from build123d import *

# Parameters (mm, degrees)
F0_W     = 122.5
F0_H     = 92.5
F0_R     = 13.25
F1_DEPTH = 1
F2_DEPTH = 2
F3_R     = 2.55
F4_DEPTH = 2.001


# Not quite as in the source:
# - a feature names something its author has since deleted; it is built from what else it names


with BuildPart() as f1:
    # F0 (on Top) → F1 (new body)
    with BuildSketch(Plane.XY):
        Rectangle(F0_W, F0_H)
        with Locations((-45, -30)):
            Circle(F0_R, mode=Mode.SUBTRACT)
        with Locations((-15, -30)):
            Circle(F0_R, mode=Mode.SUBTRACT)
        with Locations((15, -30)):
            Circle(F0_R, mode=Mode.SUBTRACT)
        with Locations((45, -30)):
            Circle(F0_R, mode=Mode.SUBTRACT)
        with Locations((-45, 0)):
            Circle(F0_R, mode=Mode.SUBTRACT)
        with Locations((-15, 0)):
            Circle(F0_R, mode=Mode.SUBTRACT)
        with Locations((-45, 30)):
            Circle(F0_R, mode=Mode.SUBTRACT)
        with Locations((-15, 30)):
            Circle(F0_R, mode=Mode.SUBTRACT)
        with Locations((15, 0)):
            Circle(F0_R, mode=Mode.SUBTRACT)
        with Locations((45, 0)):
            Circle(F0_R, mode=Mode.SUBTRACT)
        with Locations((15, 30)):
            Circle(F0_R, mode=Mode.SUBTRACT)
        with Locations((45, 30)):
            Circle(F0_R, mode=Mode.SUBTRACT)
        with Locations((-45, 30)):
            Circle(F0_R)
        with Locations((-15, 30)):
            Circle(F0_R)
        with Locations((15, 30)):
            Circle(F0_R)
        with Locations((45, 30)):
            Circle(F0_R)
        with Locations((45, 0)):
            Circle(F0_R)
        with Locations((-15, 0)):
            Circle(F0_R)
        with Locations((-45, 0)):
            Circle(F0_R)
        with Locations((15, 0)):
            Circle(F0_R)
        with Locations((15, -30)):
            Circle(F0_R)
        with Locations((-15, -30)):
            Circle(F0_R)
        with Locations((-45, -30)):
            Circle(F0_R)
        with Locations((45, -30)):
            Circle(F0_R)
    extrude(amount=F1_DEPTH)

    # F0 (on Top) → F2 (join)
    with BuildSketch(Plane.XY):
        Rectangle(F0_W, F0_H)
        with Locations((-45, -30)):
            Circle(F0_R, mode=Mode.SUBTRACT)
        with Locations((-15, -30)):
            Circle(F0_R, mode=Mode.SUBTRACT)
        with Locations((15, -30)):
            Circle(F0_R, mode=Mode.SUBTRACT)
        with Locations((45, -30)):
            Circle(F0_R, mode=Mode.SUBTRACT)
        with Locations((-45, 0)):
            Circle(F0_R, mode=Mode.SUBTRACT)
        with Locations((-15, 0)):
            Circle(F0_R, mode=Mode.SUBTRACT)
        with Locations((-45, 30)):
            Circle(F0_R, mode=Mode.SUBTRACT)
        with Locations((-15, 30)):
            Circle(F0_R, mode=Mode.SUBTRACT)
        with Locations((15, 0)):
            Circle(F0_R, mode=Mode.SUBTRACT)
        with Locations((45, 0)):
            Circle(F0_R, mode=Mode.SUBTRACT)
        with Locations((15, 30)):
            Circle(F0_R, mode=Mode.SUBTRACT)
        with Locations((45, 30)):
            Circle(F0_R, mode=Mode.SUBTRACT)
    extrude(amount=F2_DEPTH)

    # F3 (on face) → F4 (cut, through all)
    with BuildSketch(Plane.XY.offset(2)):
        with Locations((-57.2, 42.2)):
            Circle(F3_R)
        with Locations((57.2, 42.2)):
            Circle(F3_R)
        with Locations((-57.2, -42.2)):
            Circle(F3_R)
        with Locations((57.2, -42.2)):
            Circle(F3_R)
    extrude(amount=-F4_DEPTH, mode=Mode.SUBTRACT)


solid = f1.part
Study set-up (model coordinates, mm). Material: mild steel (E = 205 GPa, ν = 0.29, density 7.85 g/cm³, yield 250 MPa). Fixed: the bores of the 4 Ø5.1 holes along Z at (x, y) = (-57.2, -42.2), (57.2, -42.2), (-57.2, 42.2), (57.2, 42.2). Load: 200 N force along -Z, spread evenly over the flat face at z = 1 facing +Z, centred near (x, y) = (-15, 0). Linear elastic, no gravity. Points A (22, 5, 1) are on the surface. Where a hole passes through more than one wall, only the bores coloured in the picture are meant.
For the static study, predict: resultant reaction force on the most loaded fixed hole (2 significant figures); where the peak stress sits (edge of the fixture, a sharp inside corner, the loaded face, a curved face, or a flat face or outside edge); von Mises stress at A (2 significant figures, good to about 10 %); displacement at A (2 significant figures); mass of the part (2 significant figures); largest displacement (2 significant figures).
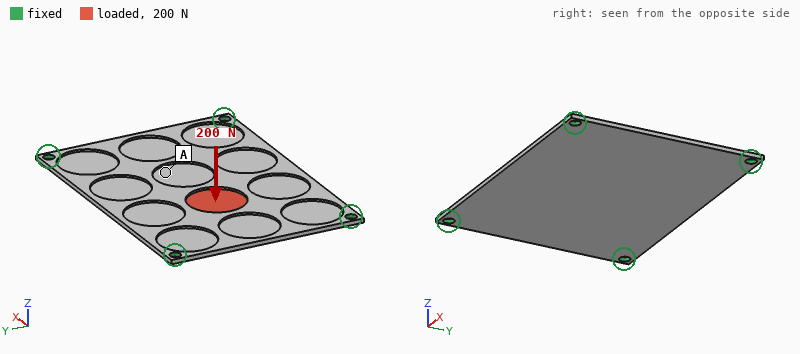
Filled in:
71 N
a curved face
22 MPa
0.33 mm
120 g
0.51 mm
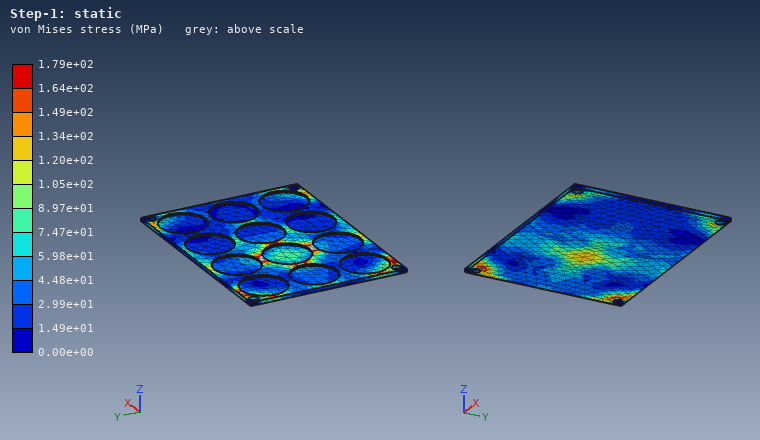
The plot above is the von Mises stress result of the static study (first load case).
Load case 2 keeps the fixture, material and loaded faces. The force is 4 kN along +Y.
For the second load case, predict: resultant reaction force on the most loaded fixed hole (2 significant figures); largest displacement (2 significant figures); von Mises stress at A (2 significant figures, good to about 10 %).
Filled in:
1.4 kN
72 µm
39 MPa
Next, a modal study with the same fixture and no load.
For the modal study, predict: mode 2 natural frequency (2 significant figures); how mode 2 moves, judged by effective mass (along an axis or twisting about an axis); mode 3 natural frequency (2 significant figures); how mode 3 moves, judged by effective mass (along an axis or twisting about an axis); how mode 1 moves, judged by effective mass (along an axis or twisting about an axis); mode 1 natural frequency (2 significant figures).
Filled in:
840 Hz
twisting about X
1100 Hz
twisting about Y
along Z
490 Hz
